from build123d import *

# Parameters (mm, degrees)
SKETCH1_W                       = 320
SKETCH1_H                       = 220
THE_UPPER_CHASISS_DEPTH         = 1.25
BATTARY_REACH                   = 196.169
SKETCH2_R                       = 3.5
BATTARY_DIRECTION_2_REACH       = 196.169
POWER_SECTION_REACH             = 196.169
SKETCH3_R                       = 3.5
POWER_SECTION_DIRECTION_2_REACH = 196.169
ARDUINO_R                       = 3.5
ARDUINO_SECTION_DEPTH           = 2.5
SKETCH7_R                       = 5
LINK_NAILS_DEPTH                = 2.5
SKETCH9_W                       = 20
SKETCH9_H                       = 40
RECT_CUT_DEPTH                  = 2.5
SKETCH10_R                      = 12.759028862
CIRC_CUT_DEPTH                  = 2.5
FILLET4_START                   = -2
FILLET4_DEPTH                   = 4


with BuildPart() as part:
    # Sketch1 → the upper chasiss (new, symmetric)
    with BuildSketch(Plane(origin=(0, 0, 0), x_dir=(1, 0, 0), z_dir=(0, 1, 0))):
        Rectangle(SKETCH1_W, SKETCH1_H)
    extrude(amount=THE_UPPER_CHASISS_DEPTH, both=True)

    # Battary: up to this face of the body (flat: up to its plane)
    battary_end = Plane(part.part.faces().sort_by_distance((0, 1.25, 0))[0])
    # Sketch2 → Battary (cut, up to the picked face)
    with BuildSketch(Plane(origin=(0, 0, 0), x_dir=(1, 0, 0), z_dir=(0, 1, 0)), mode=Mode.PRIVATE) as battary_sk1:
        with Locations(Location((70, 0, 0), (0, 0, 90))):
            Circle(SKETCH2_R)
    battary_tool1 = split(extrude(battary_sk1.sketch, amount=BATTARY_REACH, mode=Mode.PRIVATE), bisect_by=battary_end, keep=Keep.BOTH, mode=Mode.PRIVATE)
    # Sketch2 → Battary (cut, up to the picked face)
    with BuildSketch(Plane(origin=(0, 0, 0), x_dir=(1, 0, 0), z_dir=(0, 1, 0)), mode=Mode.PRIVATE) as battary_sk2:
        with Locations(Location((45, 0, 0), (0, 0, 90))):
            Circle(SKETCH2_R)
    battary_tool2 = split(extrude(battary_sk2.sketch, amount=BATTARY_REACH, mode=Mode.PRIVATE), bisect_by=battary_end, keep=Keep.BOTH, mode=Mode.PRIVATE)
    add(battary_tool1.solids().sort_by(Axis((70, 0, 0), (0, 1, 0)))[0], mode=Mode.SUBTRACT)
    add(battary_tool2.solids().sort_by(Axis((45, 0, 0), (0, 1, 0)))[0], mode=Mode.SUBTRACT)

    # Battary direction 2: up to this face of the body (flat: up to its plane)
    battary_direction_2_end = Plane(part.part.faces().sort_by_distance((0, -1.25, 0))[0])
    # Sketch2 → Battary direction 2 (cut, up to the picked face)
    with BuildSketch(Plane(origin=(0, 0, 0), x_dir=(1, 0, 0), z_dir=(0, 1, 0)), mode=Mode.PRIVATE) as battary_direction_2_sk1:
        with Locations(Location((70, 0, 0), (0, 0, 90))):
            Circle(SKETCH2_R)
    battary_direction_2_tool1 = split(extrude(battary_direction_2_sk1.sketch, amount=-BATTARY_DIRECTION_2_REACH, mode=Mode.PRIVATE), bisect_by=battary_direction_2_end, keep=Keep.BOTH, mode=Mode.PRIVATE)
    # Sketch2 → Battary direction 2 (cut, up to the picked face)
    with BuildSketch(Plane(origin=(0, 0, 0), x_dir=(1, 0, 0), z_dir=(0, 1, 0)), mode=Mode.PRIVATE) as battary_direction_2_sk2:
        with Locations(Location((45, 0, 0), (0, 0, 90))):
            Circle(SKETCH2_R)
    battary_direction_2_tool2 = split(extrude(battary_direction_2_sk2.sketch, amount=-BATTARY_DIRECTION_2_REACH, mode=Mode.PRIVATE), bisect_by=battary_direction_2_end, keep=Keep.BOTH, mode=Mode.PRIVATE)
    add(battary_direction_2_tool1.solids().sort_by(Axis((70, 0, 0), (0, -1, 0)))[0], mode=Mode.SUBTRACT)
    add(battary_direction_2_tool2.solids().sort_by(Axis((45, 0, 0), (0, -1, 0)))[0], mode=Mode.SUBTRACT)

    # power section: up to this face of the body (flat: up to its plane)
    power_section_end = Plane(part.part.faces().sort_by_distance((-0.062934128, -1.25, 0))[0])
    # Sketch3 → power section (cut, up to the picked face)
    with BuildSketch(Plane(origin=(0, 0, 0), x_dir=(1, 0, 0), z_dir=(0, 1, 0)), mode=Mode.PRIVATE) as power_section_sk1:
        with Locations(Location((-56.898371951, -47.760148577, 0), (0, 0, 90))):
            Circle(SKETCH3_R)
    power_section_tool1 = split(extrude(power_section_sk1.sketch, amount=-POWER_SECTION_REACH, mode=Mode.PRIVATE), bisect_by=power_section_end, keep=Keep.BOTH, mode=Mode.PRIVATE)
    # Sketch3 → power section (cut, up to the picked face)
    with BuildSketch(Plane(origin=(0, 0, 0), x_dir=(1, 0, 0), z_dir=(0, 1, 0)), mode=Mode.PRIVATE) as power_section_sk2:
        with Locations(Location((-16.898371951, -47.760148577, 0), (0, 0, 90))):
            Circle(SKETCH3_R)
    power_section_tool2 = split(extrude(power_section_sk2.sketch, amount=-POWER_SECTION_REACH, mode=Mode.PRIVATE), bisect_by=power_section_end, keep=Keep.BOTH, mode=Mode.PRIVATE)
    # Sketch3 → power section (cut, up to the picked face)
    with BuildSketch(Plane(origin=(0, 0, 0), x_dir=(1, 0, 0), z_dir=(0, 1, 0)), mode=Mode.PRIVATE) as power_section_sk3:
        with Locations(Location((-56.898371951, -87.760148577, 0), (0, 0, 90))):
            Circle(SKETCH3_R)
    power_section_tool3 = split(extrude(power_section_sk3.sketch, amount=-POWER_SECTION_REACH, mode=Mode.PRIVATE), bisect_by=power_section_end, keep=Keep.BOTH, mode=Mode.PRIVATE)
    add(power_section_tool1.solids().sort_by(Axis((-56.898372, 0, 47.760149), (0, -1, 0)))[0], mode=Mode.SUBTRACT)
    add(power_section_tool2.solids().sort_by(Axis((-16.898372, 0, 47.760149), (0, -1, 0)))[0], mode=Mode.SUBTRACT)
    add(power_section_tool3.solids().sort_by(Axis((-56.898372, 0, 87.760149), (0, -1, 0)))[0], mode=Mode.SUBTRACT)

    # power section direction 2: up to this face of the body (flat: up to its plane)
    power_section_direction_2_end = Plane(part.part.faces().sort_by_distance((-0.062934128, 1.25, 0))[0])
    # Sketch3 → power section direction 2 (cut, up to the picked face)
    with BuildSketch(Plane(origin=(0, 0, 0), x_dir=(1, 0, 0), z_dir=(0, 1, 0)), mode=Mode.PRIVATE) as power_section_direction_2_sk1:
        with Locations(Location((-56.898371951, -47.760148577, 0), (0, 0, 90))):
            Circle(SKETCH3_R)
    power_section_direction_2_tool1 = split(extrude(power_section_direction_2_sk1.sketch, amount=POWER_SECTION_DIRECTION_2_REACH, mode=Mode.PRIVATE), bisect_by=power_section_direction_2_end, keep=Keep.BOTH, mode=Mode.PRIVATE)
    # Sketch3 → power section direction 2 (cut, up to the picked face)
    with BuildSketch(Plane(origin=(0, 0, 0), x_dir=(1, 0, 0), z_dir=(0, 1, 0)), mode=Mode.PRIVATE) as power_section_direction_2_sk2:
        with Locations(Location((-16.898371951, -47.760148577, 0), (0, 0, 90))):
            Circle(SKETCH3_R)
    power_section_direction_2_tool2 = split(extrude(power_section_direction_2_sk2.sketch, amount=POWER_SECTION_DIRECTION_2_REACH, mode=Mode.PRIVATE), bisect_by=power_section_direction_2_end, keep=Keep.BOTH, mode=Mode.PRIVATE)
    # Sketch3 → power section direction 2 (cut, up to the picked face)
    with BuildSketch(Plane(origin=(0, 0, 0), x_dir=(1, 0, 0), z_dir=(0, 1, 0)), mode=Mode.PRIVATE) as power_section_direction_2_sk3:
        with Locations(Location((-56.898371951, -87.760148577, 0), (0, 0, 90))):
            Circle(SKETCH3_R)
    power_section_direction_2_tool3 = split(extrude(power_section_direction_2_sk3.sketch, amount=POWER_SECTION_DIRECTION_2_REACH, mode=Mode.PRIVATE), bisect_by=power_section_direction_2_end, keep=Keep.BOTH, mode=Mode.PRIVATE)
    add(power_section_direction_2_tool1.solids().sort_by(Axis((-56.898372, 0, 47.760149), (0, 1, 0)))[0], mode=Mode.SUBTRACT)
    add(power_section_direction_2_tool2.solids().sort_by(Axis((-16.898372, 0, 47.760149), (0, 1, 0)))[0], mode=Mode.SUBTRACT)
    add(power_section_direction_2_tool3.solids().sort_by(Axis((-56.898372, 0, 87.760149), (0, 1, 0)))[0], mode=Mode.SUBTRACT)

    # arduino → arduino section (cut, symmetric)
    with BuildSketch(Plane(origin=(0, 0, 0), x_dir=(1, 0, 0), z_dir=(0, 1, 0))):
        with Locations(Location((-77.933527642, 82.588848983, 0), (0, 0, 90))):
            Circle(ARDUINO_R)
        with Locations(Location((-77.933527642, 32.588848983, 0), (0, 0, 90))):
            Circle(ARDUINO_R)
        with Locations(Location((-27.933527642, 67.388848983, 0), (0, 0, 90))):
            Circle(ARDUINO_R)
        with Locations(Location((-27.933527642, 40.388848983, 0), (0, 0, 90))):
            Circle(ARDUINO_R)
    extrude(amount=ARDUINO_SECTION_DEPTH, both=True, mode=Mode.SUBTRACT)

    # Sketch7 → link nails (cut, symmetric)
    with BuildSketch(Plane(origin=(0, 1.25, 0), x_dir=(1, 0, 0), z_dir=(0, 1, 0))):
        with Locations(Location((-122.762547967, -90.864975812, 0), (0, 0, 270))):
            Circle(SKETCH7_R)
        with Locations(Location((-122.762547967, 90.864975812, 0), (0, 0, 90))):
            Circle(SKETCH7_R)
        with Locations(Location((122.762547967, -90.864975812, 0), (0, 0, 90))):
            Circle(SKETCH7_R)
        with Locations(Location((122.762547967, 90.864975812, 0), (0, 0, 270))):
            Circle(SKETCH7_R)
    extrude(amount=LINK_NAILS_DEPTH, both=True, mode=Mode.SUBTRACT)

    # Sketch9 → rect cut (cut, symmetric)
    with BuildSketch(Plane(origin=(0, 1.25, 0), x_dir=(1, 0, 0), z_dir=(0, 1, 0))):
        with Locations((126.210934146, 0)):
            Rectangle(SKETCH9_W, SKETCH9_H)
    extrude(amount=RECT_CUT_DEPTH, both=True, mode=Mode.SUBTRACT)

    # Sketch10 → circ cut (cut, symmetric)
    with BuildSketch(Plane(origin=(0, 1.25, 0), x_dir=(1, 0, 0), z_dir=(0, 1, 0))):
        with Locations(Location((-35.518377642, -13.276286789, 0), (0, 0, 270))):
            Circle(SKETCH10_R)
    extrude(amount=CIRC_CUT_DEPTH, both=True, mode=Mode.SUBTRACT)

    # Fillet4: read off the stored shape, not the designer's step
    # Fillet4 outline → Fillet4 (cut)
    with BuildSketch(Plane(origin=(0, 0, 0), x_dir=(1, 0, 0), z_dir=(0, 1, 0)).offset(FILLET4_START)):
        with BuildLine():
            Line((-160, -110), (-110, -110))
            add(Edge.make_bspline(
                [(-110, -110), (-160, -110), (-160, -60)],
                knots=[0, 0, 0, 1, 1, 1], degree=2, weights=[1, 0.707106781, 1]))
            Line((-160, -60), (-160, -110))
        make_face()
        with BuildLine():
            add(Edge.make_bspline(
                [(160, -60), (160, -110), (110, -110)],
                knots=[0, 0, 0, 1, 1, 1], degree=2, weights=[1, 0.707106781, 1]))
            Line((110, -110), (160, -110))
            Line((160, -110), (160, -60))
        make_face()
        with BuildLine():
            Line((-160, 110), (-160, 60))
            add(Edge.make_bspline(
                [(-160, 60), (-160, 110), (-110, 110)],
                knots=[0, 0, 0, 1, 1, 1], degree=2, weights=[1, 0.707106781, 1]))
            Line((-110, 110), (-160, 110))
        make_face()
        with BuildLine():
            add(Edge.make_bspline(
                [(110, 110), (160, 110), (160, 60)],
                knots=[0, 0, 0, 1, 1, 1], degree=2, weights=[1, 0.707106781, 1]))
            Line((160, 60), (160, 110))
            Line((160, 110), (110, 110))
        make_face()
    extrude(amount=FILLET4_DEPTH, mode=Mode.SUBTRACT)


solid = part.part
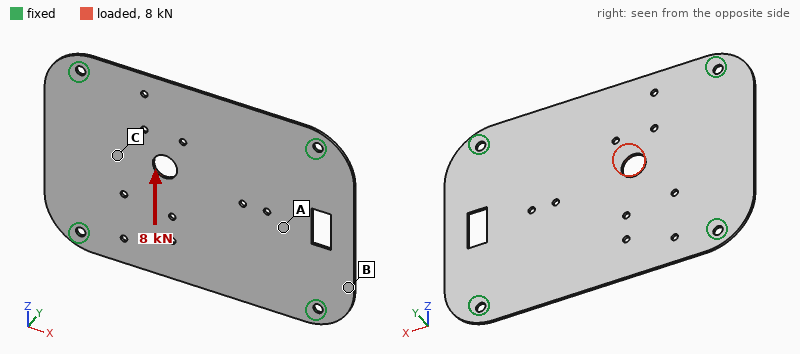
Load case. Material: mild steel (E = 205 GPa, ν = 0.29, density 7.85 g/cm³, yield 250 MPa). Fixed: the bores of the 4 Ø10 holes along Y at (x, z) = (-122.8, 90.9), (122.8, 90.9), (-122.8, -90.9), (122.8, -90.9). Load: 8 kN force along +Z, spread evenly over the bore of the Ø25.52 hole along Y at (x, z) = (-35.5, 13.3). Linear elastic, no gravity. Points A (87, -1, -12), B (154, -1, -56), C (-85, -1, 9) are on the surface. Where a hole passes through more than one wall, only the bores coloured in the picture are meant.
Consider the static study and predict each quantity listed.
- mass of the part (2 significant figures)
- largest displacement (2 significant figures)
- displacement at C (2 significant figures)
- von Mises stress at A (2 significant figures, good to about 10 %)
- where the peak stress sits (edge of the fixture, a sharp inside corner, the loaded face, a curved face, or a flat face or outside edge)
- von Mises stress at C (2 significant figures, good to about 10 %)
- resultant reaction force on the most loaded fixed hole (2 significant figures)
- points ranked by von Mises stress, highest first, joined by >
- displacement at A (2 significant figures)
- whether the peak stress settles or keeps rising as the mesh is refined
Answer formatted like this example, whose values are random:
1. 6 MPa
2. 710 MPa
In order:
1. 1.3 kg
2. 20 µm
3. 9.3 µm
4. 10 MPa
5. edge of the fixture
6. 18 MPa
7. 2.9 kN
8. C > A > B
9. 5.2 µm
10. keeps rising
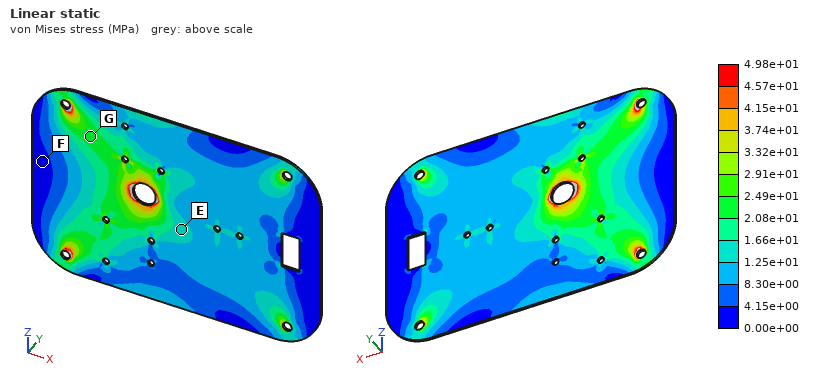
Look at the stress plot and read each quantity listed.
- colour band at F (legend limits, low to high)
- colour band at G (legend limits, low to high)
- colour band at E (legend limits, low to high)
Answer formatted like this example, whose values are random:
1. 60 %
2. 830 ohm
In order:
1. 0.00e+00 to 4.15e+00 MPa
2. 2.08e+01 to 2.49e+01 MPa
3. 1.25e+01 to 1.66e+01 MPa
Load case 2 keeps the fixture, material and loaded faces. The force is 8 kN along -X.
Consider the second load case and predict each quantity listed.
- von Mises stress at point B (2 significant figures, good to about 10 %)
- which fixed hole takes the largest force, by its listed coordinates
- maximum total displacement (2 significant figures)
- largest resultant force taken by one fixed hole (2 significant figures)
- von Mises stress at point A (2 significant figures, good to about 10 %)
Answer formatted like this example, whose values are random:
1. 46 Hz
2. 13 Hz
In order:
1. 4.3 MPa
2. (-122.8, 90.9)
3. 15 µm
4. 2.6 kN
5. 4.5 MPa
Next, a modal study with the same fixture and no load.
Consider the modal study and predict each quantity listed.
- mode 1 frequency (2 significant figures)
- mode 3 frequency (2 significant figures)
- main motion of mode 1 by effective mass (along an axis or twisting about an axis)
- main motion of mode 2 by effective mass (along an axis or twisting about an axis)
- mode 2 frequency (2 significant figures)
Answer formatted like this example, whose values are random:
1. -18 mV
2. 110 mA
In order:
1. 180 Hz
2. 380 Hz
3. along Y
4. twisting about X
5. 280 Hz
